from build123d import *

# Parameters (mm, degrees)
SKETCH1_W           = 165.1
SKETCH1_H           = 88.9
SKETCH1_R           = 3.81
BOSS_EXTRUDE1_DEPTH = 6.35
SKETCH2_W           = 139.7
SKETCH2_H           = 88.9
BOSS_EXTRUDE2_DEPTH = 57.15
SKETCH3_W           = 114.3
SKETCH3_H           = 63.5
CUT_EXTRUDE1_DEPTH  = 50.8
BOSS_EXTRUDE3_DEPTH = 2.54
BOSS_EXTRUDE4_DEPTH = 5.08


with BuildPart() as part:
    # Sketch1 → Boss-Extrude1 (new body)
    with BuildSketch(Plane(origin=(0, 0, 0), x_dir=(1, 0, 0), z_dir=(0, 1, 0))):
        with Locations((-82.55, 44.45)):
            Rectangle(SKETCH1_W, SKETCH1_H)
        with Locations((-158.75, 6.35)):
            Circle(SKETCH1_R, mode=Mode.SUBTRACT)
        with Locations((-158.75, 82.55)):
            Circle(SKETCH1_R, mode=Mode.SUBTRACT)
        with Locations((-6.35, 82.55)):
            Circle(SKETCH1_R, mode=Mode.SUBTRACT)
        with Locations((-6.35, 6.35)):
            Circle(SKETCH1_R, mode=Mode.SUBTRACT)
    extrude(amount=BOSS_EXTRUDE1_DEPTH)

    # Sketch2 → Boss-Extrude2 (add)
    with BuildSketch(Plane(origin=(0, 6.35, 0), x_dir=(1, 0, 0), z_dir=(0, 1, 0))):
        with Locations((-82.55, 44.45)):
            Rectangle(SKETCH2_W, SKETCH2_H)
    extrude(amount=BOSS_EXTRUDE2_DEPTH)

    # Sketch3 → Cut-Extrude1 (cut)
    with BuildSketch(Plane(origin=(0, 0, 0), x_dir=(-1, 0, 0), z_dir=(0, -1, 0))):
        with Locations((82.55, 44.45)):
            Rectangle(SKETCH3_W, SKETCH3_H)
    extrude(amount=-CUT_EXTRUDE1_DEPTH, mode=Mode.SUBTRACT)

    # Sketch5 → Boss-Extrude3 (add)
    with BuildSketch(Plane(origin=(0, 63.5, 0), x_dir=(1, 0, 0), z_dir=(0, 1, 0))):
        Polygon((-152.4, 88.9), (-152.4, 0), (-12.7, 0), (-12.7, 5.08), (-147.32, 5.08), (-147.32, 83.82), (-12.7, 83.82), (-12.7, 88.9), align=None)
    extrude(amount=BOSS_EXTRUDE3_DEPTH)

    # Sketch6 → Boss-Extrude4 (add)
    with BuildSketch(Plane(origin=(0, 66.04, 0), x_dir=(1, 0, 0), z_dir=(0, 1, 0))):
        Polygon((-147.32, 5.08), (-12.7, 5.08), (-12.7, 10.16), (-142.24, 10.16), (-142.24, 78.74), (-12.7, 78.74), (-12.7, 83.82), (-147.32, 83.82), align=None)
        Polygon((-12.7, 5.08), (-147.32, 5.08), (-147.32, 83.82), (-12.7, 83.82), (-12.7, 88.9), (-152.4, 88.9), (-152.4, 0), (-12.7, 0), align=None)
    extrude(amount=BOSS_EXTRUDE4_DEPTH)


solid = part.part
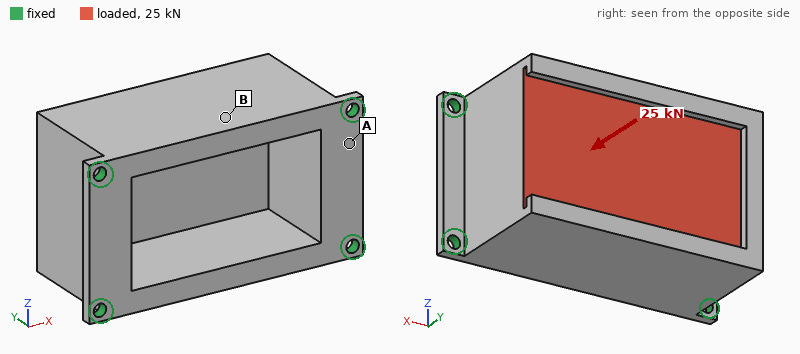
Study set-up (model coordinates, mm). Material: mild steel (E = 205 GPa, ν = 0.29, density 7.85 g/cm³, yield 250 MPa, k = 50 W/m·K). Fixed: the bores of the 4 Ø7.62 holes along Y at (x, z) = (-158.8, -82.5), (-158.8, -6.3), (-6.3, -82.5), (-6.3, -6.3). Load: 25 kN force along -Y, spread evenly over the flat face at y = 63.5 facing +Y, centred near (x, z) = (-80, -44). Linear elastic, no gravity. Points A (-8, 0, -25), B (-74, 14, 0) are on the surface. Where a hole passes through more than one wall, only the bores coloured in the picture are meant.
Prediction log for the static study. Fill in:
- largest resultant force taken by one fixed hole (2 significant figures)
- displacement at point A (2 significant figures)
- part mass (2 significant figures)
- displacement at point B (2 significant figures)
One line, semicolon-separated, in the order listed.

7.4 kN; 8.6 µm; 3.6 kg; 15 µm
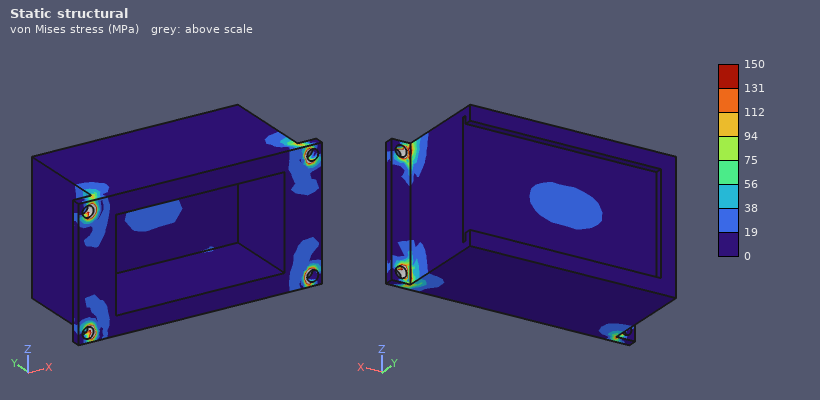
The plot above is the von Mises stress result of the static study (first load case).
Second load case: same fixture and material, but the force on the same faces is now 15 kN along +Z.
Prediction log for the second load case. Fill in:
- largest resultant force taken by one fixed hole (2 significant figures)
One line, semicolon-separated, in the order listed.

7.6 kN
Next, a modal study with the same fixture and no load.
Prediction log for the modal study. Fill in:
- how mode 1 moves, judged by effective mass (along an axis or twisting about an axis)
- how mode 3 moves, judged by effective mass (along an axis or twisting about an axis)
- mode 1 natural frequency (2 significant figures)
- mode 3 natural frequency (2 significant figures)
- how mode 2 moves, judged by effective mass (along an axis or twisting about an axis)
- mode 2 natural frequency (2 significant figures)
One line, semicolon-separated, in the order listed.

along Z; along X; 2600 Hz; 4200 Hz; along Y; 3800 Hz
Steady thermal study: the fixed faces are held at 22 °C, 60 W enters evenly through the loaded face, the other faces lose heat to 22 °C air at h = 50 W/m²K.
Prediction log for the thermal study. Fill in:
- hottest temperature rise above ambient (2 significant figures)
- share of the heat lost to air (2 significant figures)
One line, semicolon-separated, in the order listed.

20 K; 69 %
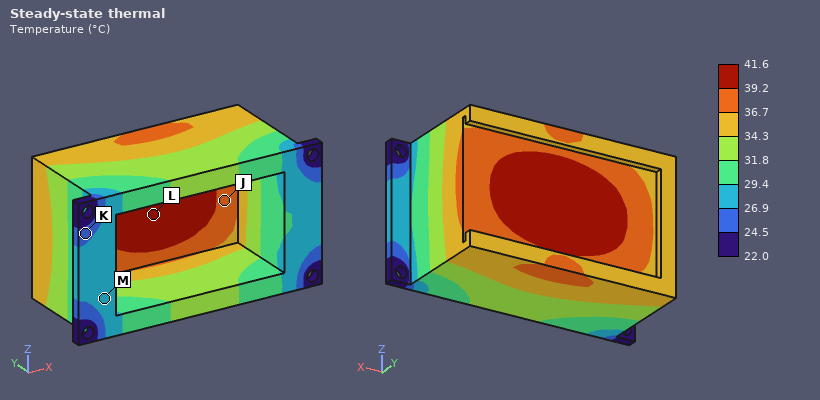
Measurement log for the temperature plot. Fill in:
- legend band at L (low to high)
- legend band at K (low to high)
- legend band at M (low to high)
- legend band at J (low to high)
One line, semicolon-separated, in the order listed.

39.2 to 41.6 °C; 24.5 to 26.9 °C; 26.9 to 29.4 °C; 36.7 to 39.2 °C
